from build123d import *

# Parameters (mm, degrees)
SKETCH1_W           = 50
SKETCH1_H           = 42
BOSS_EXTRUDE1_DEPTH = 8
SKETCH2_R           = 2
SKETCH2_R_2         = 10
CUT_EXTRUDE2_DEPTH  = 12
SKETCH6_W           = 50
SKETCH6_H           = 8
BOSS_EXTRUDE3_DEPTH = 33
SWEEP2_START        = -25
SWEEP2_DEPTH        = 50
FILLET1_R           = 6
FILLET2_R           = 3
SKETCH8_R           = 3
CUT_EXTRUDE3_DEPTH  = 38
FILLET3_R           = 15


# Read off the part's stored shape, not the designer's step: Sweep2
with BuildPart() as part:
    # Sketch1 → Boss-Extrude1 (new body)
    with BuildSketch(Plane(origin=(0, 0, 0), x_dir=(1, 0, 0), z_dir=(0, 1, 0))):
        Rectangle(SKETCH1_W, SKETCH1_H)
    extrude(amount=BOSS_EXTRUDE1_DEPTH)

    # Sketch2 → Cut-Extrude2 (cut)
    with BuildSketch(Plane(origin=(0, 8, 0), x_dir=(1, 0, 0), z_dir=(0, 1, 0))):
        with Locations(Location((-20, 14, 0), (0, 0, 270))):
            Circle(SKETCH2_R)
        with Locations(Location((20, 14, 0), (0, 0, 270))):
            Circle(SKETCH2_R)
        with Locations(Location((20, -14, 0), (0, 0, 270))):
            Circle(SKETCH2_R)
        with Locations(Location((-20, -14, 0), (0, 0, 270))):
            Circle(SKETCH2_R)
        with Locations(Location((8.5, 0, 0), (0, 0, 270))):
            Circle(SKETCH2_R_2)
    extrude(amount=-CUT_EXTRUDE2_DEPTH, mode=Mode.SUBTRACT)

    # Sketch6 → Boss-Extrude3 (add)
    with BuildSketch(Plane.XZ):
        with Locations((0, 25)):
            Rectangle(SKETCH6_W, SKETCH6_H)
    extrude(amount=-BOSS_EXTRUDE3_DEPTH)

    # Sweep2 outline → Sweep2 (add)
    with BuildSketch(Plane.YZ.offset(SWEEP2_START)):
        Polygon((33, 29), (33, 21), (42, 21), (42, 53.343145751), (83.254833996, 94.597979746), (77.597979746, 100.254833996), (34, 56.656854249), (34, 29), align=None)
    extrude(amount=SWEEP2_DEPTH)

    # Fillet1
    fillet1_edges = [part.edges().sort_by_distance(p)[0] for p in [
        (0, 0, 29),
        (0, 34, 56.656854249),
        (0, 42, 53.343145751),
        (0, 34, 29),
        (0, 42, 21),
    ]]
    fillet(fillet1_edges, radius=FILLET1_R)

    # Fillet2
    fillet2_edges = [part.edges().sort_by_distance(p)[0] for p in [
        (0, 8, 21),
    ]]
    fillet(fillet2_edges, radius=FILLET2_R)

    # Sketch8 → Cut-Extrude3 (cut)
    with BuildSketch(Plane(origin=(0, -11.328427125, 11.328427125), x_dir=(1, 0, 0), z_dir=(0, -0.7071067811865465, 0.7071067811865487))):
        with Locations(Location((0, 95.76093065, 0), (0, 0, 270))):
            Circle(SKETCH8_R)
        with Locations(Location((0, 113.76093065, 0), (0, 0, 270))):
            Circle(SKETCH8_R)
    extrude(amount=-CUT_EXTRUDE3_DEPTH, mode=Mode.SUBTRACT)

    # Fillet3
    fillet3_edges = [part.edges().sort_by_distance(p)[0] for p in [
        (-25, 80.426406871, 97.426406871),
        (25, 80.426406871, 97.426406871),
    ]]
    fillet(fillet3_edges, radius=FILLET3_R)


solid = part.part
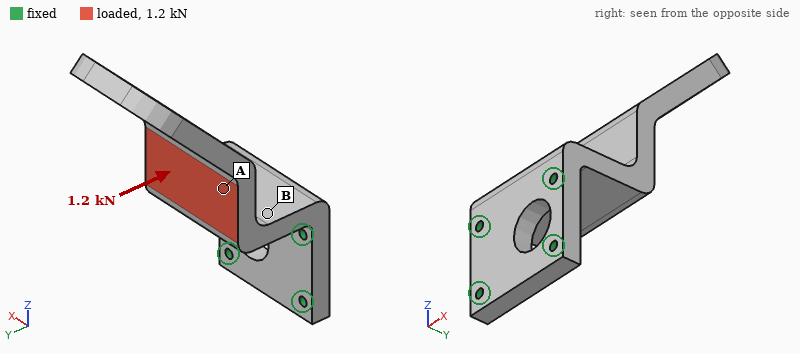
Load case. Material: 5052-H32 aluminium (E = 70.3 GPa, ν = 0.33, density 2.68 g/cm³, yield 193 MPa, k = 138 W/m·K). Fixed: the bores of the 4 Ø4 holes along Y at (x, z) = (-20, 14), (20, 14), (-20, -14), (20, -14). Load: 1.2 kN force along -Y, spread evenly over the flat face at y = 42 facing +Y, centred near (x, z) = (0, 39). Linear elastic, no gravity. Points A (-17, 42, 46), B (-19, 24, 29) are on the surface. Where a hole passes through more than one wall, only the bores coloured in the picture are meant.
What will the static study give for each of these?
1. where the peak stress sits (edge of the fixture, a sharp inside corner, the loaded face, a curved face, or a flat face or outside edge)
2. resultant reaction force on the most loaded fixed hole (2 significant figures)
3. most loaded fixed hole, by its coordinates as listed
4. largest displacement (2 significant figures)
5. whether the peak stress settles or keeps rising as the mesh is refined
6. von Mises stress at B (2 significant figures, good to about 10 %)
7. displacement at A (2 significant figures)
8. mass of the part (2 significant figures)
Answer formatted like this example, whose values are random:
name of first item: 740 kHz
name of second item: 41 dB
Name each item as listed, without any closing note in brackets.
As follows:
where the peak stress sits: edge of the fixture
resultant reaction force on the most loaded fixed hole: 800 N
most loaded fixed hole, by its coordinates as listed: (-20, 14)
largest displacement: 0.53 mm
whether the peak stress settles or keeps rising as the mesh is refined: keeps rising
von Mises stress at B: 34 MPa
displacement at A: 0.19 mm
mass of the part: 170 g
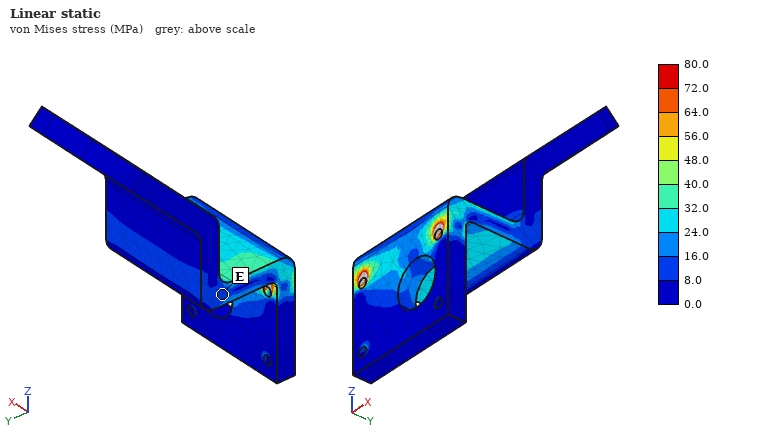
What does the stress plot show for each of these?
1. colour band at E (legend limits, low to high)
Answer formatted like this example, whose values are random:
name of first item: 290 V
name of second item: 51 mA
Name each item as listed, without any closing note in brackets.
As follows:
colour band at E: 8.0 to 16.0 MPa
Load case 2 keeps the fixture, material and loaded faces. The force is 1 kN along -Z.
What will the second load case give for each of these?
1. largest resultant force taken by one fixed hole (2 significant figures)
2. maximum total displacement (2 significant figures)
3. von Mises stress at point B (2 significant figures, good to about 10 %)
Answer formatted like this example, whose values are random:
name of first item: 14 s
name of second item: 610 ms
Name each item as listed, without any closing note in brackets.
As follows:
largest resultant force taken by one fixed hole: 480 N
maximum total displacement: 0.70 mm
von Mises stress at point B: 35 MPa
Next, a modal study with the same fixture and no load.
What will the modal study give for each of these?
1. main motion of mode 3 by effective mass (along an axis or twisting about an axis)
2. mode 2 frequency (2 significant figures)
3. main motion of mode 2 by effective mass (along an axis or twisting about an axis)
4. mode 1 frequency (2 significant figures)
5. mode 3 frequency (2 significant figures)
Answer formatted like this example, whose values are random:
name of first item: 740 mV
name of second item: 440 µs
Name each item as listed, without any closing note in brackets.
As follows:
main motion of mode 3 by effective mass: along Z
mode 2 frequency: 1300 Hz
main motion of mode 2 by effective mass: along X
mode 1 frequency: 490 Hz
mode 3 frequency: 2600 Hz
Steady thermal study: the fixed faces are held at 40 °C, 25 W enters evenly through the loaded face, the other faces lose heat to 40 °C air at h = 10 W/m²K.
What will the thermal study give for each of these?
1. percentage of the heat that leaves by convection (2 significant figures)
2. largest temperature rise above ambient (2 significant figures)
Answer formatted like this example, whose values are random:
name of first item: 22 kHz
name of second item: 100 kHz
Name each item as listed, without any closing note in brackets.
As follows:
percentage of the heat that leaves by convection: 9.8 %
largest temperature rise above ambient: 22 K
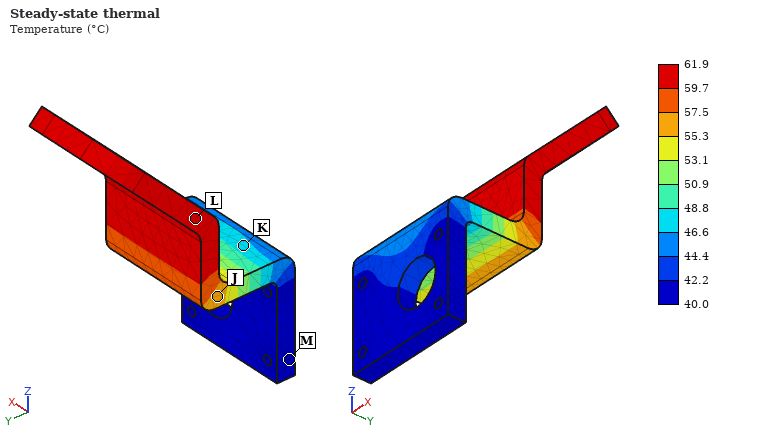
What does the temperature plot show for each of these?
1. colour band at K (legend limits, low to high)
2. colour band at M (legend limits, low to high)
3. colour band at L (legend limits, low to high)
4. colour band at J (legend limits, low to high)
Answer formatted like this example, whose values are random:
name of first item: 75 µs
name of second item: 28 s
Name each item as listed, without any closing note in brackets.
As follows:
colour band at K: 46.6 to 48.8 °C
colour band at M: 40.0 to 42.2 °C
colour band at L: 59.7 to 61.9 °C
colour band at J: 55.3 to 57.5 °C
